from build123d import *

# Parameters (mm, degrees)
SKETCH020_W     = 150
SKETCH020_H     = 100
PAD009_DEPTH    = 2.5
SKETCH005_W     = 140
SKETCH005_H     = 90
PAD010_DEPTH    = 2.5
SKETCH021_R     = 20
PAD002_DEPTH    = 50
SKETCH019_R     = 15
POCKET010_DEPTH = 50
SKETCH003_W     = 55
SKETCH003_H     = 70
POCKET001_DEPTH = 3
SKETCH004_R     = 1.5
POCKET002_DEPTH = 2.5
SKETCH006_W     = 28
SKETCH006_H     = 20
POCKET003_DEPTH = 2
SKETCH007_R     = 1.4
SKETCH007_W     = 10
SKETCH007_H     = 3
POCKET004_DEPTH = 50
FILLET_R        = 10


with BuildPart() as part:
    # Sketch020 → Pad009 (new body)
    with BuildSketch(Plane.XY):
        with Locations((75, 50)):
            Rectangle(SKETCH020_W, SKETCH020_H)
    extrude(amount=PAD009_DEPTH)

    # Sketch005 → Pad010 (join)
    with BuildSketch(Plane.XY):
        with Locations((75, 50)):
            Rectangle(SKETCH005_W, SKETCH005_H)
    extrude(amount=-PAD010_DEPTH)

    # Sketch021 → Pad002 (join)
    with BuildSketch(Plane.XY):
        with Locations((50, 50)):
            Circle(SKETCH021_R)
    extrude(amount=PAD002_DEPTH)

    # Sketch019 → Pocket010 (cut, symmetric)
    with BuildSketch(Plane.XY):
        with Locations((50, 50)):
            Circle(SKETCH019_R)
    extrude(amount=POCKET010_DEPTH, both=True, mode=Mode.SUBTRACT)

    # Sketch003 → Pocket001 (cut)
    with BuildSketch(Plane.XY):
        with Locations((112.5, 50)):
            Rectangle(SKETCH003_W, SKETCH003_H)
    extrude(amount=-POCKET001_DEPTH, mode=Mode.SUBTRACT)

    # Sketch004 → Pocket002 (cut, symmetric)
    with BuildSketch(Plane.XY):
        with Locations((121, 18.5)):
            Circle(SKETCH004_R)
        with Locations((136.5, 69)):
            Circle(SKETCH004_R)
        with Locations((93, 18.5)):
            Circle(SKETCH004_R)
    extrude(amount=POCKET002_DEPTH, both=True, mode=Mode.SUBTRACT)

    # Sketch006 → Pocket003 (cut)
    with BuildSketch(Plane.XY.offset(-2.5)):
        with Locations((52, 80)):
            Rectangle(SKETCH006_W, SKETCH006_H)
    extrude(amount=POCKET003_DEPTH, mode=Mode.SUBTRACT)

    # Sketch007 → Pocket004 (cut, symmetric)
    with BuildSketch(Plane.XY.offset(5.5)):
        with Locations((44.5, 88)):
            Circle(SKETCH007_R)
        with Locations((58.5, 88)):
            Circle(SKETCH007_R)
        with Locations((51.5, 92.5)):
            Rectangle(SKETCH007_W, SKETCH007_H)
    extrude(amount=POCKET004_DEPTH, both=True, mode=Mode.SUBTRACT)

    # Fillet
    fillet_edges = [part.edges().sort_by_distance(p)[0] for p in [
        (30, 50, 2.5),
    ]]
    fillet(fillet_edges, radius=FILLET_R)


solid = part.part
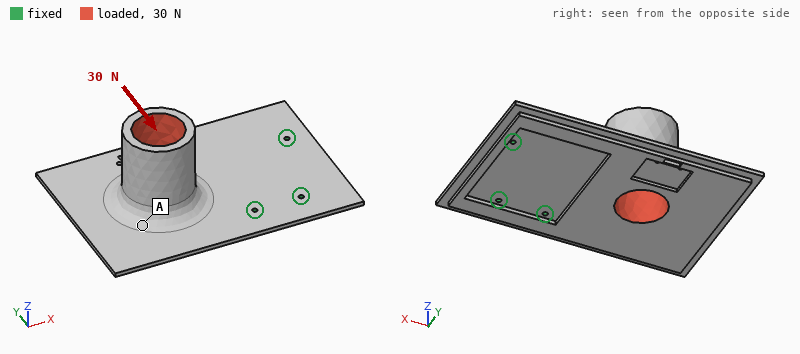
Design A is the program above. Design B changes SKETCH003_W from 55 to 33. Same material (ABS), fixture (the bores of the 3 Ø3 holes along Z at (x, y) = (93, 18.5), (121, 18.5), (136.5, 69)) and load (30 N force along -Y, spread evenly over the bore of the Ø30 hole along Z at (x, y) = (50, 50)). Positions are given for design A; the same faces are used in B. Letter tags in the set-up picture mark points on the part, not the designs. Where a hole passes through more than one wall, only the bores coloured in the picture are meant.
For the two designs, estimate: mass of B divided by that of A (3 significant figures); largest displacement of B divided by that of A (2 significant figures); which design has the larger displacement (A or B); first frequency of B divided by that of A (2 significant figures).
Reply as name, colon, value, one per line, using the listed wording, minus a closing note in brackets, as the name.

mass of B divided by that of A: 1.05
largest displacement of B divided by that of A: 0.56
which design has the larger displacement: A
first frequency of B divided by that of A: 1.4
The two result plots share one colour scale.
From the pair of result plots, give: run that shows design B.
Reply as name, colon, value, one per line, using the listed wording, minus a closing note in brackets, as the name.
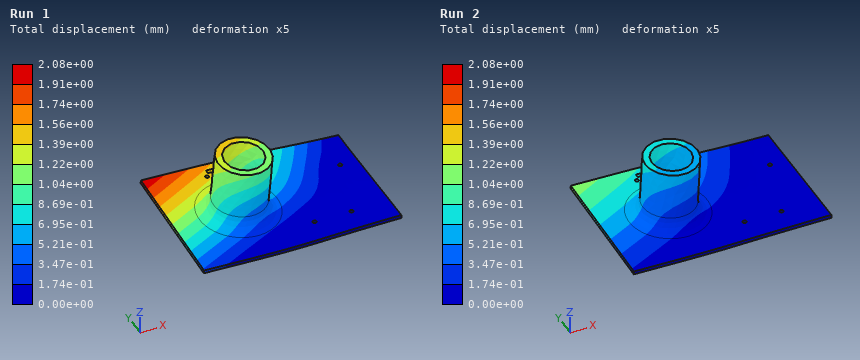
run that shows design B: Run 2
